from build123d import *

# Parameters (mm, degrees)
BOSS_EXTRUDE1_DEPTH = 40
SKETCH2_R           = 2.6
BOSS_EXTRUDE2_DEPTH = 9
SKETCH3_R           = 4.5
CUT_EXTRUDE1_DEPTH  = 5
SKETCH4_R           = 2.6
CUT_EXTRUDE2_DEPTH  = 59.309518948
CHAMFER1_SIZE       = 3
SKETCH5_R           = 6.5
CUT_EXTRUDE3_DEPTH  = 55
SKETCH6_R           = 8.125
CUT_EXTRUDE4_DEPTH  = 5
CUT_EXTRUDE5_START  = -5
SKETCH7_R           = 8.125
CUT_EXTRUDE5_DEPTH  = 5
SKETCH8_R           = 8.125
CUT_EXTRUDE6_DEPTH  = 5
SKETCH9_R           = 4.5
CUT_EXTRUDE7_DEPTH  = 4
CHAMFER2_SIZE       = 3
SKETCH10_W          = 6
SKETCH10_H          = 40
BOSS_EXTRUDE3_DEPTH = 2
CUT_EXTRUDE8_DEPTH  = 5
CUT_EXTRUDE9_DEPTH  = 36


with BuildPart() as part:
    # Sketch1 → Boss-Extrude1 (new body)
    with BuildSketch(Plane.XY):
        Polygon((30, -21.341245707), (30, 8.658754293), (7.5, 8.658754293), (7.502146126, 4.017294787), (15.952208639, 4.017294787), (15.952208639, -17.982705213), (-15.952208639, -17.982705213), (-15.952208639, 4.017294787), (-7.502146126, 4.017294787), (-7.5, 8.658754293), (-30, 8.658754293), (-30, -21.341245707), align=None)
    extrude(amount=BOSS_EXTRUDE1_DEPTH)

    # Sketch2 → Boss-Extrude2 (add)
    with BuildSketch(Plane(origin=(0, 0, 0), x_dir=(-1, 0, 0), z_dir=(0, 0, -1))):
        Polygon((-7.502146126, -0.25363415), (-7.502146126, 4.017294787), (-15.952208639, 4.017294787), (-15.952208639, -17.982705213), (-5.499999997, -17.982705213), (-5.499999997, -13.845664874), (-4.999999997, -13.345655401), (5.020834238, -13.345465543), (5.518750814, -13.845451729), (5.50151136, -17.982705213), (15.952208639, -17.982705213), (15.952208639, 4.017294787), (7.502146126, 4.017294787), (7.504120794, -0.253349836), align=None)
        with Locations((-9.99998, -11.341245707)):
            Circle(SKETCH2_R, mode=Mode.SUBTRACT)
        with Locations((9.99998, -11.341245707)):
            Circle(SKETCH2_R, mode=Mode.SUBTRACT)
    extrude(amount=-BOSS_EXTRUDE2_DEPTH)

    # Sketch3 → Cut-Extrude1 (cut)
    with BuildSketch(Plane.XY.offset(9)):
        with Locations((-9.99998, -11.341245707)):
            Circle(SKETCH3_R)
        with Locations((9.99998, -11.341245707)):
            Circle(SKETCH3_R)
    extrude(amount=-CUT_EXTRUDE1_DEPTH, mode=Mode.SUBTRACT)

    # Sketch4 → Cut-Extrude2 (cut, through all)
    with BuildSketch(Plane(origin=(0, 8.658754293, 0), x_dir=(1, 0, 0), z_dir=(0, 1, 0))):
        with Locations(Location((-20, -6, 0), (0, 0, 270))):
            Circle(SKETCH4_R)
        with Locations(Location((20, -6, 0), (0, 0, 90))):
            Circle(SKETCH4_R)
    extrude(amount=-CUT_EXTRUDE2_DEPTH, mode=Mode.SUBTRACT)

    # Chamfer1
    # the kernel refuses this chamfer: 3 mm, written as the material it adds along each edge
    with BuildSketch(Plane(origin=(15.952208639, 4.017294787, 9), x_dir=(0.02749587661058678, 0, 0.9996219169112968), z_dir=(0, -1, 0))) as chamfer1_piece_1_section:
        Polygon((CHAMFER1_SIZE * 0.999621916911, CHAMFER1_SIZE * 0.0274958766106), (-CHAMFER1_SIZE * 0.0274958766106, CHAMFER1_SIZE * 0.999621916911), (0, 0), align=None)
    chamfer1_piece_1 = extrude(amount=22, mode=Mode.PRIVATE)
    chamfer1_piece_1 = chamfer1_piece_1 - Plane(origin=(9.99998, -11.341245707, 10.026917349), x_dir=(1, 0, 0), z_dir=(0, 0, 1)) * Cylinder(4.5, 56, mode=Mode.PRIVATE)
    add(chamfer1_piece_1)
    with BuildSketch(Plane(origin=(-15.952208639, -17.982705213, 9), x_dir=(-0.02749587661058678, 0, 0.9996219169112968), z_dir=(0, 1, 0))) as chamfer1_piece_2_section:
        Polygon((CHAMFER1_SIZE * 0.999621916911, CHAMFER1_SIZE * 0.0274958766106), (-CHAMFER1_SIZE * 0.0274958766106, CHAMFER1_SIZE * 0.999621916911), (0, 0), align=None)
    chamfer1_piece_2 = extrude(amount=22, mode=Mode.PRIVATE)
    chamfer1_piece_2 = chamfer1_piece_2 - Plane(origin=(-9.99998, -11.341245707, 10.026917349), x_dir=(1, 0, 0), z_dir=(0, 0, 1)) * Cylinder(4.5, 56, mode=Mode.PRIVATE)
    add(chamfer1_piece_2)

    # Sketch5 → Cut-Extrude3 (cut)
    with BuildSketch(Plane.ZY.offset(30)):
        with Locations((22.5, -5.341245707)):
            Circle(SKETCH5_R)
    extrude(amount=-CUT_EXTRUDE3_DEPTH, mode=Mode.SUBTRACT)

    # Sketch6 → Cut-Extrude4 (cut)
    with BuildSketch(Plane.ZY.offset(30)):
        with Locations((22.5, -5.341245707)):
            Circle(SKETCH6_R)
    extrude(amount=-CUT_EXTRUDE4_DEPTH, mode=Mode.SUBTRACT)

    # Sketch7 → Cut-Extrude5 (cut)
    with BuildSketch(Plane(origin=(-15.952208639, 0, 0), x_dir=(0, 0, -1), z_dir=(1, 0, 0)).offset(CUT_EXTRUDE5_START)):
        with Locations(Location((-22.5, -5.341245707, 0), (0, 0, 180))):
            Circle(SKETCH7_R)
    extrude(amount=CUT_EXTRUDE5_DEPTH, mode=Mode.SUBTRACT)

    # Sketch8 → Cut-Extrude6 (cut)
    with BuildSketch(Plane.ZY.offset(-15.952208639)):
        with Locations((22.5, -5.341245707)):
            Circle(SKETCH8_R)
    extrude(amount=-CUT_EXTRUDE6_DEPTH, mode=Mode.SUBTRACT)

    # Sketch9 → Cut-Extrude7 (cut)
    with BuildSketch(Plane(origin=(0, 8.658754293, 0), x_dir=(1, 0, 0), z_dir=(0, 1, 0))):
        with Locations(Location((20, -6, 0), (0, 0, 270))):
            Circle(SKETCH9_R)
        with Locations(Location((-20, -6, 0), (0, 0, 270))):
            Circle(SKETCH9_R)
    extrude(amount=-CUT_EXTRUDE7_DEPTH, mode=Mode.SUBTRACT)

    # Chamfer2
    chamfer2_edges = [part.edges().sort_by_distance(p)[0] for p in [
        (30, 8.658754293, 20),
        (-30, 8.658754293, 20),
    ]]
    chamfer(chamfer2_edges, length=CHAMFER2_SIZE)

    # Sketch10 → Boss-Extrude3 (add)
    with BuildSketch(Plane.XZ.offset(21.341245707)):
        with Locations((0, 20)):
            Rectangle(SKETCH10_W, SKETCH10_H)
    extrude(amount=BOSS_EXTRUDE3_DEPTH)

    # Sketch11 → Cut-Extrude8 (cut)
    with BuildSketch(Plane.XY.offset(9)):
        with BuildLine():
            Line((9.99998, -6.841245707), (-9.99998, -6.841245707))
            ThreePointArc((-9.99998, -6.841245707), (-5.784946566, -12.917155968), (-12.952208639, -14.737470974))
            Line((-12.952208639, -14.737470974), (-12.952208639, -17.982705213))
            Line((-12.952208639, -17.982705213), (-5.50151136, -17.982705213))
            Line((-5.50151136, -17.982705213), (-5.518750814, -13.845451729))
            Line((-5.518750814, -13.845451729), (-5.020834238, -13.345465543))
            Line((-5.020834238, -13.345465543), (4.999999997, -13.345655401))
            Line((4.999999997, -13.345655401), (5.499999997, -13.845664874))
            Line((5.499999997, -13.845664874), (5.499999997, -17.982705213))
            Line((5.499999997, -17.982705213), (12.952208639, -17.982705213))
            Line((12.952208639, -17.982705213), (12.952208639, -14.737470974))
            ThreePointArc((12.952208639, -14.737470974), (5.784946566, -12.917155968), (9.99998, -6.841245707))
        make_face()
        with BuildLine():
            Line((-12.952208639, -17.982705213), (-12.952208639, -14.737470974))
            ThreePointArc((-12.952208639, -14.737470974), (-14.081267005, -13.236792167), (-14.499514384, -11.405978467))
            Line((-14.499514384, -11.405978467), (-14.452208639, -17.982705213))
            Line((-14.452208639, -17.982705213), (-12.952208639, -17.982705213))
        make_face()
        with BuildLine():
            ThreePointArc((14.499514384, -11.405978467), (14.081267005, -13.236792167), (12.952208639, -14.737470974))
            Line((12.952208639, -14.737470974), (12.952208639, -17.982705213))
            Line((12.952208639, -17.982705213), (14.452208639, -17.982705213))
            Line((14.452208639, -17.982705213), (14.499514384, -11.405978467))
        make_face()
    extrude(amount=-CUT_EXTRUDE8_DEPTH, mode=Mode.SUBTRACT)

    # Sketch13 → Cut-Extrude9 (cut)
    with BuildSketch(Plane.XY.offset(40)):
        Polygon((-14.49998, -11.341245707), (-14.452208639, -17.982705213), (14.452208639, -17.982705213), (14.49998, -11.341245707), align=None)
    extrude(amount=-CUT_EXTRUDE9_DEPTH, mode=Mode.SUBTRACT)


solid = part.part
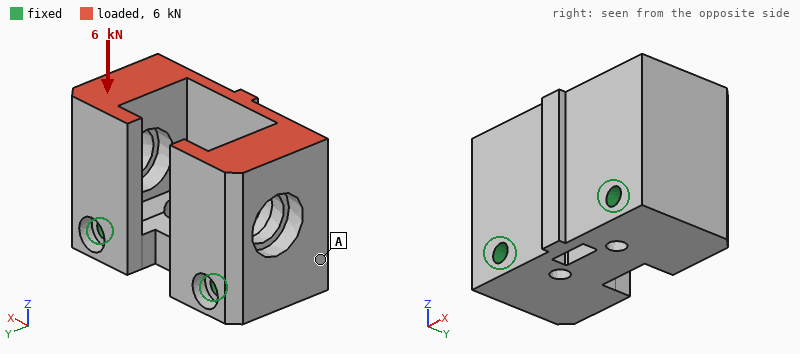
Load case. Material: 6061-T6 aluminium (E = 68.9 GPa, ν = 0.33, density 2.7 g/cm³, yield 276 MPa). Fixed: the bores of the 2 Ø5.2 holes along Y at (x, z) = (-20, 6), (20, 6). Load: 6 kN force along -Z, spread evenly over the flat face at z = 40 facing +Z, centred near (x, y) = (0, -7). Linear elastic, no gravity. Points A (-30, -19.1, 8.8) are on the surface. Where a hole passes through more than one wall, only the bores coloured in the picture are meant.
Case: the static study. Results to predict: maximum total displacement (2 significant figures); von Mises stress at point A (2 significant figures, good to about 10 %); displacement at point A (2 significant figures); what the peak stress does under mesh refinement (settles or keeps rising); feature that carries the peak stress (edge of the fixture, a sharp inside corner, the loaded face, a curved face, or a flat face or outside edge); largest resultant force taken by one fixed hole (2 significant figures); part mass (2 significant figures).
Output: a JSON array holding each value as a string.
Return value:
["8.1 µm", "4.2 MPa", "1.6 µm", "keeps rising", "edge of the fixture", "3.0 kN", "110 g"]
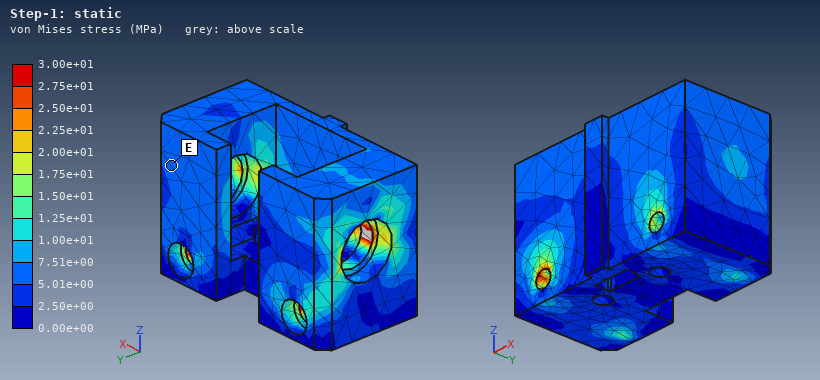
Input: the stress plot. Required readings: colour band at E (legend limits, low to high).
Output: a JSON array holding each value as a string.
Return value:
["5.01e+00 to 7.51e+00 MPa"]
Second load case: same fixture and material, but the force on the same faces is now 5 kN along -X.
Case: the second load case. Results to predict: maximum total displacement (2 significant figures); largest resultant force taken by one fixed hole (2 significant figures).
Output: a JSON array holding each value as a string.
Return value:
["71 µm", "3.6 kN"]
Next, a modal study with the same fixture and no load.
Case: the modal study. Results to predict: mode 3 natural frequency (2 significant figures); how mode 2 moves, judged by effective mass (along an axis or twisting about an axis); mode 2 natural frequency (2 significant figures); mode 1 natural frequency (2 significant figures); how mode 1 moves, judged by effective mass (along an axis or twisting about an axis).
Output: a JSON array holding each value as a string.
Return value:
["10000 Hz", "along X", "9400 Hz", "8300 Hz", "along Y"]
